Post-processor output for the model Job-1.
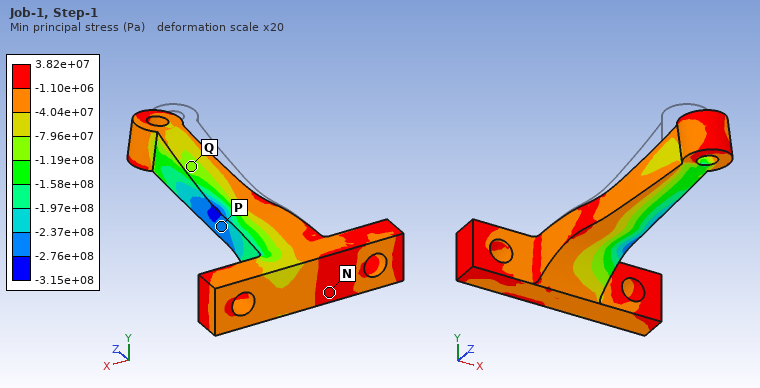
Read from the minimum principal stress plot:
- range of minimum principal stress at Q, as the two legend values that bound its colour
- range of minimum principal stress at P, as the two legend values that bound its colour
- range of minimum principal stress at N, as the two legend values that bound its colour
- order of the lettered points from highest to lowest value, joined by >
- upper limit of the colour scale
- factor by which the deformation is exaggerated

-1.19e+08 to -7.96e+07 Pa
-2.76e+08 to -2.37e+08 Pa
-1.10e+06 to 3.82e+07 Pa
N > Q > P
3.82e+07 Pa
20
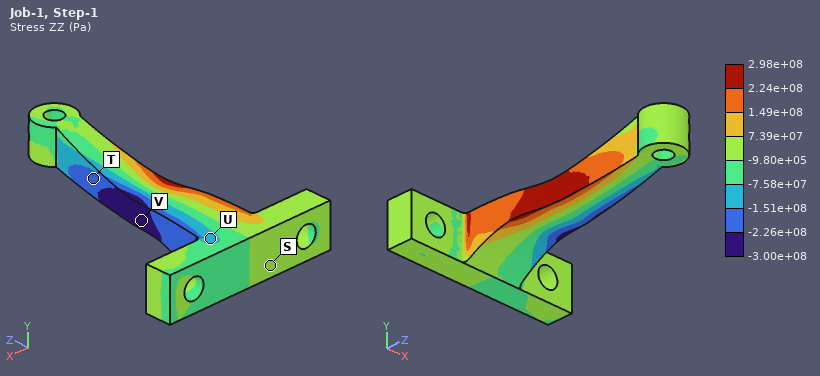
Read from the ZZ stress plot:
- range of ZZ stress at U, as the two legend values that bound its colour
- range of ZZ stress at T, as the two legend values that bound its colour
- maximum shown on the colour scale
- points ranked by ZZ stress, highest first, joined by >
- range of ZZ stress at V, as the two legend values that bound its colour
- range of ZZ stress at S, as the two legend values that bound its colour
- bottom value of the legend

-1.51e+08 to -7.58e+07 Pa
-2.26e+08 to -1.51e+08 Pa
2.98e+08 Pa
S > U > T > V
-3.00e+08 to -2.26e+08 Pa
-9.80e+05 to 7.39e+07 Pa
-3.00e+08 Pa
